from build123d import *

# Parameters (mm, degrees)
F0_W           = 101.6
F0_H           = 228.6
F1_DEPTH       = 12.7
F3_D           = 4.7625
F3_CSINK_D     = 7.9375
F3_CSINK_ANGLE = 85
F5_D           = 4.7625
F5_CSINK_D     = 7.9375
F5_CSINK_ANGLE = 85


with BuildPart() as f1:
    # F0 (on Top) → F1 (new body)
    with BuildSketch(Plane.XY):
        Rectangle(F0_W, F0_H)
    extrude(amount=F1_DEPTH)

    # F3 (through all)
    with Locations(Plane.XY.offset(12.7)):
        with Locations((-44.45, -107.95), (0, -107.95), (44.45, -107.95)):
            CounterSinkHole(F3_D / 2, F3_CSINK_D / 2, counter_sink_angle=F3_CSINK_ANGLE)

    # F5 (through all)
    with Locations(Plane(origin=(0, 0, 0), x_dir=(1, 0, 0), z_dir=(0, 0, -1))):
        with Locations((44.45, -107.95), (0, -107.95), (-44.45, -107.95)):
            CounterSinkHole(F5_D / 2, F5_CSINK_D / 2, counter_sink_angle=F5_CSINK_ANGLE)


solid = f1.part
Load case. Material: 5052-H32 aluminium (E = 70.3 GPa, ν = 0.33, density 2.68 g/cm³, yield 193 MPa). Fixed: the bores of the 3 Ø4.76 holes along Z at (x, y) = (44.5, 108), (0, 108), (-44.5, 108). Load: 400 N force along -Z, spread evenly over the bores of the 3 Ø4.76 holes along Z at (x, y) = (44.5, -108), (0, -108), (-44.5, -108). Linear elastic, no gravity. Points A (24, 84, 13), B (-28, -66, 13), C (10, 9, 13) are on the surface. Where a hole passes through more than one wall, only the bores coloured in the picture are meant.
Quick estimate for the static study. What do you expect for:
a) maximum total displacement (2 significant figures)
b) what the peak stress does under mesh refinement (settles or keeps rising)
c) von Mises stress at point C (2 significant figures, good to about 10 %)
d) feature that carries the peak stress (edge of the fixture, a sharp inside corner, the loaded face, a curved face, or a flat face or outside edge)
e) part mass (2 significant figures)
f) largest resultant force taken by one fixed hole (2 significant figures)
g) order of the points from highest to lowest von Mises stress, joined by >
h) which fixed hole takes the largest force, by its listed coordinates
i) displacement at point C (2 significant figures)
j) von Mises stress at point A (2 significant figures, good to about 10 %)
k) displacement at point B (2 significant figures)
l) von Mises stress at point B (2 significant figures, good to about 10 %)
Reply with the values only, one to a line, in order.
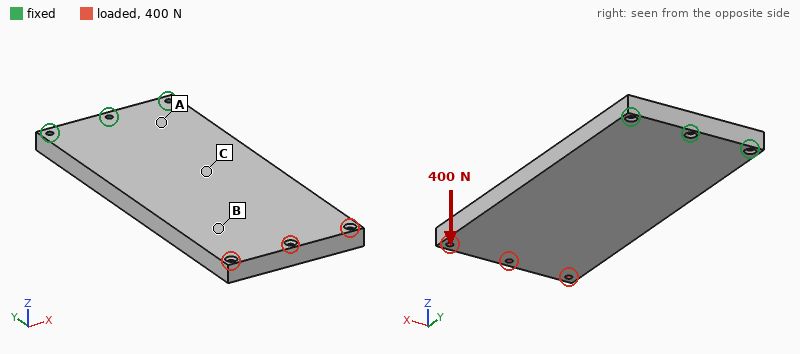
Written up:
1.3 mm
keeps rising
17 MPa
edge of the fixture
790 g
560 N
A > C > B
(0, 108)
0.37 mm
26 MPa
0.91 mm
6.3 MPa
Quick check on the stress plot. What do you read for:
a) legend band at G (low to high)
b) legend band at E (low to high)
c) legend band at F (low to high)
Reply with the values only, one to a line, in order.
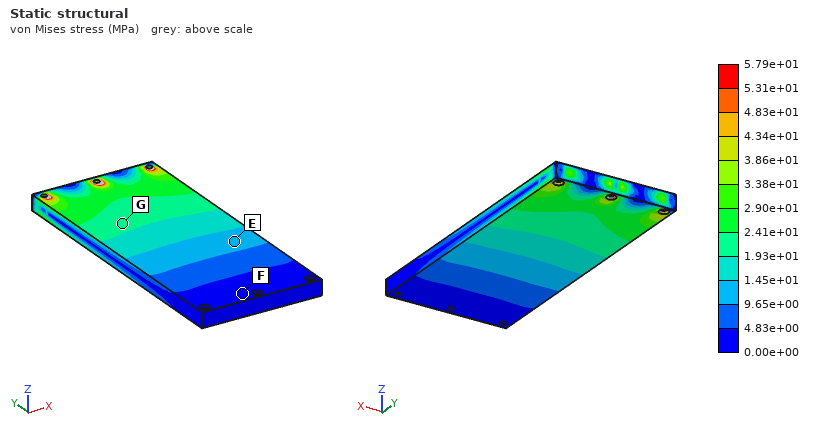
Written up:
1.93e+01 to 2.41e+01 MPa
9.65e+00 to 1.45e+01 MPa
0.00e+00 to 4.83e+00 MPa
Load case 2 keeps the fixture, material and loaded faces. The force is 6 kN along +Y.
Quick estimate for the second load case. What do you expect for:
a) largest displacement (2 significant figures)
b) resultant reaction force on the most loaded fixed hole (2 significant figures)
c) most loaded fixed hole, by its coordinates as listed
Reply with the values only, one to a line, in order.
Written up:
0.12 mm
2.3 kN
(0, 108)
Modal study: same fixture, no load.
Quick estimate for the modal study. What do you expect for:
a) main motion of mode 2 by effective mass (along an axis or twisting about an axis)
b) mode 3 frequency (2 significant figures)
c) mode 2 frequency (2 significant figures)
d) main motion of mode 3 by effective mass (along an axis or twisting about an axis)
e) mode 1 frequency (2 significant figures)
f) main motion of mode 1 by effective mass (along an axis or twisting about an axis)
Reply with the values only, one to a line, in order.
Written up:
twisting about Y
1200 Hz
940 Hz
along Z
200 Hz
along Z
